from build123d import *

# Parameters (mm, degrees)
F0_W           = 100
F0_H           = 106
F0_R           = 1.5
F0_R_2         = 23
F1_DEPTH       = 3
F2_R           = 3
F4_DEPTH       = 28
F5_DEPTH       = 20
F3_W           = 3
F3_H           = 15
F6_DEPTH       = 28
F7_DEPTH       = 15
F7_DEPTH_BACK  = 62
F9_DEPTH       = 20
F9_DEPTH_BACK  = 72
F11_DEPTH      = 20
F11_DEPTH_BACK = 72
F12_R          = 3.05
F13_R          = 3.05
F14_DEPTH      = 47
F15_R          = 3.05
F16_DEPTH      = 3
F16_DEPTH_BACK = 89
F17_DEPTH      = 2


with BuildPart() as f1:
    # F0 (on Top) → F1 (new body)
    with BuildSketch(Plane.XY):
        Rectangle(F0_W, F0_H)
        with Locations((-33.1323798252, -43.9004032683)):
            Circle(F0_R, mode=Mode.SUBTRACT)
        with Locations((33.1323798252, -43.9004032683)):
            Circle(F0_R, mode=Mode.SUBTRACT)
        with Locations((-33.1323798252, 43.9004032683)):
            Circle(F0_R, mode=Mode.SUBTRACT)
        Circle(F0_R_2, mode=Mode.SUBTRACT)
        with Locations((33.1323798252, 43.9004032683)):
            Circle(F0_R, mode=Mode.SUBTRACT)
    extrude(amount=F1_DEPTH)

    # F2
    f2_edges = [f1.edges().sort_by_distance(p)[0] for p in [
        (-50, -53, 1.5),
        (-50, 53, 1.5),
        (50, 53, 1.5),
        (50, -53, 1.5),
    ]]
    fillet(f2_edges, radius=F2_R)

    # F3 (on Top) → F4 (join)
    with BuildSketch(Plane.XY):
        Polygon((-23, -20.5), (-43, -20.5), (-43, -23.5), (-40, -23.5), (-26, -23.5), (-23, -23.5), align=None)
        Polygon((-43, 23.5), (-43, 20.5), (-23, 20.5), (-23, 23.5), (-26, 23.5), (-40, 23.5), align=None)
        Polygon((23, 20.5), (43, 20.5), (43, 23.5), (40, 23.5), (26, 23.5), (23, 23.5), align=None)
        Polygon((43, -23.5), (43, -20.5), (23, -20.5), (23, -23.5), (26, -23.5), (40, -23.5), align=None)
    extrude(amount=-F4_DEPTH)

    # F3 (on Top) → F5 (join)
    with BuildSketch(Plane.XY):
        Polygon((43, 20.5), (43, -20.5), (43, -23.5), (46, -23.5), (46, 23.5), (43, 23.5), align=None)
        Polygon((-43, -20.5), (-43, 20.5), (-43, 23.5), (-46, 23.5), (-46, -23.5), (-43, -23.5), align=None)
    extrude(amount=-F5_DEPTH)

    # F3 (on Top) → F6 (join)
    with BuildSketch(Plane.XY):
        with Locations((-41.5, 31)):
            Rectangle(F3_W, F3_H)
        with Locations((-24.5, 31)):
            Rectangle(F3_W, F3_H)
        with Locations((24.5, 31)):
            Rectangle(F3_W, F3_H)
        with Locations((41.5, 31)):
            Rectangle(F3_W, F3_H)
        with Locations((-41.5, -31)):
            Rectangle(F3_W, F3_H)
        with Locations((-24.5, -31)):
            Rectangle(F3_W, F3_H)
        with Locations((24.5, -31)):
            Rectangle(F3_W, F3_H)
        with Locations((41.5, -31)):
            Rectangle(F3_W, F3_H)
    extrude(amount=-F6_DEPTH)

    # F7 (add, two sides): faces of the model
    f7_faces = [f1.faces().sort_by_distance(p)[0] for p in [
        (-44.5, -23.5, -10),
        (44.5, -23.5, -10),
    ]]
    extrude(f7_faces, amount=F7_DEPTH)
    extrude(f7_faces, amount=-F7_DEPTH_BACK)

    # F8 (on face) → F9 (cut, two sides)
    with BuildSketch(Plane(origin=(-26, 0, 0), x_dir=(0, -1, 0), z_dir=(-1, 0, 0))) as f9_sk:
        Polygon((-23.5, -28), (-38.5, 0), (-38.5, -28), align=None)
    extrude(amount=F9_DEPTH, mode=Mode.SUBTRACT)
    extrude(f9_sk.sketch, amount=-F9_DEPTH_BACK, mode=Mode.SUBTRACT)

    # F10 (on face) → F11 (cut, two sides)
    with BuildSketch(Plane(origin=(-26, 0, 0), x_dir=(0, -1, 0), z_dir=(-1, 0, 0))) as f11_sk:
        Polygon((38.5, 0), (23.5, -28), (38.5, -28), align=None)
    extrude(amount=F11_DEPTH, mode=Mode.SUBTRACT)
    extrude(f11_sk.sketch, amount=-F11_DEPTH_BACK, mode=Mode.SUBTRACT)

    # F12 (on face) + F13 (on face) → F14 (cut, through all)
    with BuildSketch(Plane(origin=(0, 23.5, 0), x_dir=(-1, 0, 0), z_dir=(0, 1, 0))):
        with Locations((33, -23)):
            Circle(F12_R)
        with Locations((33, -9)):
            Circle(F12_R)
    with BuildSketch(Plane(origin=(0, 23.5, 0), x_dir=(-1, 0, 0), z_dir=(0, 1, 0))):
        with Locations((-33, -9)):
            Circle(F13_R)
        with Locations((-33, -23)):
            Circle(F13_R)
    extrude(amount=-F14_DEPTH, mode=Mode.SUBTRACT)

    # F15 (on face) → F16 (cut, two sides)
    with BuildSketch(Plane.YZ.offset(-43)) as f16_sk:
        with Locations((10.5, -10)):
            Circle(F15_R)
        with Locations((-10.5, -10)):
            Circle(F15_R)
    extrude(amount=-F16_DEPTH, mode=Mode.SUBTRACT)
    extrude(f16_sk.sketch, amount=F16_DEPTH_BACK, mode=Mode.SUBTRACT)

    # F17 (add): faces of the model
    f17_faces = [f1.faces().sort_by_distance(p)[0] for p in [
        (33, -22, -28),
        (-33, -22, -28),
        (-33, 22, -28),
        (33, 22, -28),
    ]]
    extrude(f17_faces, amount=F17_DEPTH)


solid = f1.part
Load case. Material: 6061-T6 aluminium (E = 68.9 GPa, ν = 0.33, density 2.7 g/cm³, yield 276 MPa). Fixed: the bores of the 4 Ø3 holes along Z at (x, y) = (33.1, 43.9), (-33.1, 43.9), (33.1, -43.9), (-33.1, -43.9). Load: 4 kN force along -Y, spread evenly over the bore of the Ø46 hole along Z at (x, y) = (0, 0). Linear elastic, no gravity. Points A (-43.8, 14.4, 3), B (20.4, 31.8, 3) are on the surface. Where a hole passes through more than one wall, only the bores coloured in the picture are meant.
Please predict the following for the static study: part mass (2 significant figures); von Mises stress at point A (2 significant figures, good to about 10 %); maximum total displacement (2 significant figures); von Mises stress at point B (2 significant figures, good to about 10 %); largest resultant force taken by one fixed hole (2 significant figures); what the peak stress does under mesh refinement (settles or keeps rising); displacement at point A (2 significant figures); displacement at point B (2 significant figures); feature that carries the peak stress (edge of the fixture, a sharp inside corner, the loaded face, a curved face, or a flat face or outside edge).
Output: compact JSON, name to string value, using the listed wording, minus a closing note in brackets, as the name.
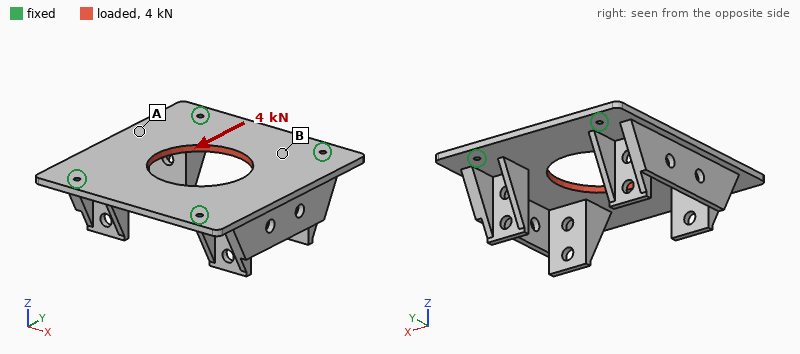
{"part mass": "120 g", "von Mises stress at point A": "3.4 MPa", "maximum total displacement": "11 µm", "von Mises stress at point B": "13 MPa", "largest resultant force taken by one fixed hole": "1.0 kN", "what the peak stress does under mesh refinement": "keeps rising", "displacement at point A": "4.2 µm", "displacement at point B": "6.4 µm", "feature that carries the peak stress": "edge of the fixture"}
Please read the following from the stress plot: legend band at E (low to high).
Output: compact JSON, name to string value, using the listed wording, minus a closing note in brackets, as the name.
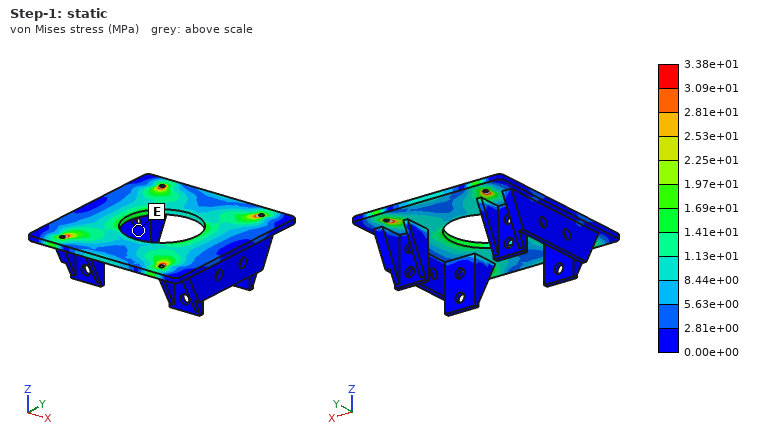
{"legend band at E": "0.00e+00 to 2.81e+00 MPa"}
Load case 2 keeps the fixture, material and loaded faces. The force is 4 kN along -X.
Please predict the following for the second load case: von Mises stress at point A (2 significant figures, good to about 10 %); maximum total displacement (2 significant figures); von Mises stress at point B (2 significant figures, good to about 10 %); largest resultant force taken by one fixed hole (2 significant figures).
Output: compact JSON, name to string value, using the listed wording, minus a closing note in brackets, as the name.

{"von Mises stress at point A": "9.6 MPa", "maximum total displacement": "18 µm", "von Mises stress at point B": "13 MPa", "largest resultant force taken by one fixed hole": "1.0 kN"}
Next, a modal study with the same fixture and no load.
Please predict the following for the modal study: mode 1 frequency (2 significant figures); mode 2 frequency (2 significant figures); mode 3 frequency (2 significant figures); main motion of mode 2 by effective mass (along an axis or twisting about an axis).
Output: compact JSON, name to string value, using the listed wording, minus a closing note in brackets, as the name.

{"mode 1 frequency": "1800 Hz", "mode 2 frequency": "2600 Hz", "mode 3 frequency": "2700 Hz", "main motion of mode 2 by effective mass": "along X"}
